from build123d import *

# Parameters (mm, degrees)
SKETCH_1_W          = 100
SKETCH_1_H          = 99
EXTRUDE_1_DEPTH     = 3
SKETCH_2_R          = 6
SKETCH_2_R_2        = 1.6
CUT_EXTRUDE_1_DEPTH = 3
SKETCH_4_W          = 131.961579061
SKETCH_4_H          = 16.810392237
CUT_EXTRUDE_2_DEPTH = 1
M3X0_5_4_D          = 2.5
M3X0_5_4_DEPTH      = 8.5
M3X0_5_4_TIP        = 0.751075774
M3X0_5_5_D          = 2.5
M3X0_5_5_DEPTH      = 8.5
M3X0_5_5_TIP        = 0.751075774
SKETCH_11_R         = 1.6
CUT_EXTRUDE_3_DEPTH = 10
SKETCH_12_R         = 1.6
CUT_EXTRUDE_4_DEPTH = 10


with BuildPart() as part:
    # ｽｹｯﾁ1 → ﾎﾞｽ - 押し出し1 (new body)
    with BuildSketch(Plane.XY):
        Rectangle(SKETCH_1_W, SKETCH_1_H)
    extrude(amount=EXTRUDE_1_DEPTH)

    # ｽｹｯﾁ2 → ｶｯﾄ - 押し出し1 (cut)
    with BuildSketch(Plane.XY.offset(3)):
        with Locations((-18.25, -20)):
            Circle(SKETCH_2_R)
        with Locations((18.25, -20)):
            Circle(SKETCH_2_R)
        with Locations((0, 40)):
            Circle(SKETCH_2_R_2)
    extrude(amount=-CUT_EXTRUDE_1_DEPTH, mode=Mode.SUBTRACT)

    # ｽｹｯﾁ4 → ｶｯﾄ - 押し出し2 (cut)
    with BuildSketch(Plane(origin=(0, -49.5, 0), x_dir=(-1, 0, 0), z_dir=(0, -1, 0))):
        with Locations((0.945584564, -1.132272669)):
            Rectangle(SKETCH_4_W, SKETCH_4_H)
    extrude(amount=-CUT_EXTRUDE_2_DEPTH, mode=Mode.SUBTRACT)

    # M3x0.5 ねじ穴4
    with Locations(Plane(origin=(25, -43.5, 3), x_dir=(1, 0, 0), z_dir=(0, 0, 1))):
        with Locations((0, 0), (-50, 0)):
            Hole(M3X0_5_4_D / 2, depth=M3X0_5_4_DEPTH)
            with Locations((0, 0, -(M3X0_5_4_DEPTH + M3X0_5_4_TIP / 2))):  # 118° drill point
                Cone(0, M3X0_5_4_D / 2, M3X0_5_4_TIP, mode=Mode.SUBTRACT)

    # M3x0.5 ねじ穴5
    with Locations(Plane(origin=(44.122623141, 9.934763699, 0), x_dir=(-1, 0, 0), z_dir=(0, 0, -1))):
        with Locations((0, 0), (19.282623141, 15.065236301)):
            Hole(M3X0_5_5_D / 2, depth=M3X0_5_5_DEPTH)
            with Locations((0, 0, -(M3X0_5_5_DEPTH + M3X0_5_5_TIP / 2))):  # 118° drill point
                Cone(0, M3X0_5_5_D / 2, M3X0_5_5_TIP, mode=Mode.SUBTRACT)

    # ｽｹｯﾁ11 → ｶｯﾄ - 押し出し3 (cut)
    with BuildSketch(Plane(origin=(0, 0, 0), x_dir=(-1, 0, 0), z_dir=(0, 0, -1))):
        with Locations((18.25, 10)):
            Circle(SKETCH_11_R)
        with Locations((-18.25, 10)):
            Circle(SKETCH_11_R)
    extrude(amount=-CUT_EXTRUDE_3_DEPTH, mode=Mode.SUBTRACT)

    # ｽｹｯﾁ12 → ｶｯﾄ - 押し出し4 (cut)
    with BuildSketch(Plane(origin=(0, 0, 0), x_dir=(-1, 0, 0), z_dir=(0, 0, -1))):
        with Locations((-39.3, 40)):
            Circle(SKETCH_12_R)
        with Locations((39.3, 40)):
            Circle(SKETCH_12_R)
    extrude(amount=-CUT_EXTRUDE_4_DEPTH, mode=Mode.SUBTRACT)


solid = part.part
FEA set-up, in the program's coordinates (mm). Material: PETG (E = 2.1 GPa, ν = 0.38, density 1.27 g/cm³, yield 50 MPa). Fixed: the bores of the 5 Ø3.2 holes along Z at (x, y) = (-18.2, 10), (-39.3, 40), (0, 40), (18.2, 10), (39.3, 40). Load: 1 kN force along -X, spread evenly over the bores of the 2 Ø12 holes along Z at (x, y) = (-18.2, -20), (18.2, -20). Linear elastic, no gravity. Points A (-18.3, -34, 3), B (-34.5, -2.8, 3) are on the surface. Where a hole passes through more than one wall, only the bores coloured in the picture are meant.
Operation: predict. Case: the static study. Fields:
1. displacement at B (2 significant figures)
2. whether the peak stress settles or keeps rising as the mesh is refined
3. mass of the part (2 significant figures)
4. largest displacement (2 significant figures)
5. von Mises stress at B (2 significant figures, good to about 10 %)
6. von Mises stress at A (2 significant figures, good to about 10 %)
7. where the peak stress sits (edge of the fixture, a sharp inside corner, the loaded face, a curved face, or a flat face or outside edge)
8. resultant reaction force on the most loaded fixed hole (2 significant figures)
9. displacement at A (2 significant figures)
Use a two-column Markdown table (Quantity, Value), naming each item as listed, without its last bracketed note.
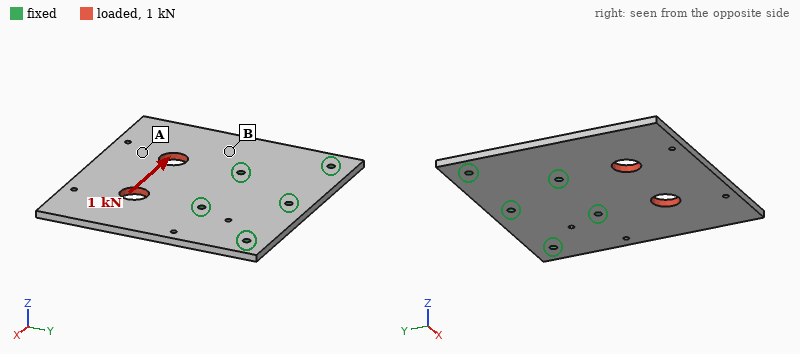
| Quantity | Value |
|---|---|
| displacement at B | 0.15 mm |
| whether the peak stress settles or keeps rising as the mesh is refined | keeps rising |
| mass of the part | 36 g |
| largest displacement | 0.39 mm |
| von Mises stress at B | 5.0 MPa |
| von Mises stress at A | 2.0 MPa |
| where the peak stress sits | edge of the fixture |
| resultant reaction force on the most loaded fixed hole | 560 N |
| displacement at A | 0.32 mm |
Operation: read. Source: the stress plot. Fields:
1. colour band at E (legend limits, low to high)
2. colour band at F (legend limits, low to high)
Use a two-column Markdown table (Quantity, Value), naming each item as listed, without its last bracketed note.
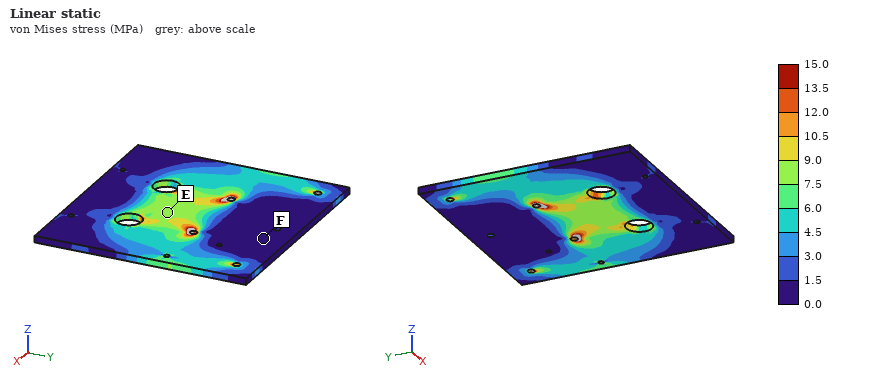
| Quantity | Value |
|---|---|
| colour band at E | 7.5 to 9.0 MPa |
| colour band at F | 0.0 to 1.5 MPa |
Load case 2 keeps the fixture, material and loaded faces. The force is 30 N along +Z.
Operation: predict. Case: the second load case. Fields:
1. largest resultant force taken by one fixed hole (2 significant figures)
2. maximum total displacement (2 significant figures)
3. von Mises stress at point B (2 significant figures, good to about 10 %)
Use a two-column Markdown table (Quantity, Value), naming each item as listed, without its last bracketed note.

| Quantity | Value |
|---|---|
| largest resultant force taken by one fixed hole | 23 N |
| maximum total displacement | 1.7 mm |
| von Mises stress at point B | 3.0 MPa |
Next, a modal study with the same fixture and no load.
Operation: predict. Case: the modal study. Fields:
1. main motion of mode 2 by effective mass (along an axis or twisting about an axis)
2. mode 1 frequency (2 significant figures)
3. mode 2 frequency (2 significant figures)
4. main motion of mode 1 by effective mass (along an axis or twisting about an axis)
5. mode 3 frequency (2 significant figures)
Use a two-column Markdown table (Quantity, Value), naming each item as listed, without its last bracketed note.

| Quantity | Value |
|---|---|
| main motion of mode 2 by effective mass | twisting about Y |
| mode 1 frequency | 170 Hz |
| mode 2 frequency | 250 Hz |
| main motion of mode 1 by effective mass | along Z |
| mode 3 frequency | 500 Hz |
